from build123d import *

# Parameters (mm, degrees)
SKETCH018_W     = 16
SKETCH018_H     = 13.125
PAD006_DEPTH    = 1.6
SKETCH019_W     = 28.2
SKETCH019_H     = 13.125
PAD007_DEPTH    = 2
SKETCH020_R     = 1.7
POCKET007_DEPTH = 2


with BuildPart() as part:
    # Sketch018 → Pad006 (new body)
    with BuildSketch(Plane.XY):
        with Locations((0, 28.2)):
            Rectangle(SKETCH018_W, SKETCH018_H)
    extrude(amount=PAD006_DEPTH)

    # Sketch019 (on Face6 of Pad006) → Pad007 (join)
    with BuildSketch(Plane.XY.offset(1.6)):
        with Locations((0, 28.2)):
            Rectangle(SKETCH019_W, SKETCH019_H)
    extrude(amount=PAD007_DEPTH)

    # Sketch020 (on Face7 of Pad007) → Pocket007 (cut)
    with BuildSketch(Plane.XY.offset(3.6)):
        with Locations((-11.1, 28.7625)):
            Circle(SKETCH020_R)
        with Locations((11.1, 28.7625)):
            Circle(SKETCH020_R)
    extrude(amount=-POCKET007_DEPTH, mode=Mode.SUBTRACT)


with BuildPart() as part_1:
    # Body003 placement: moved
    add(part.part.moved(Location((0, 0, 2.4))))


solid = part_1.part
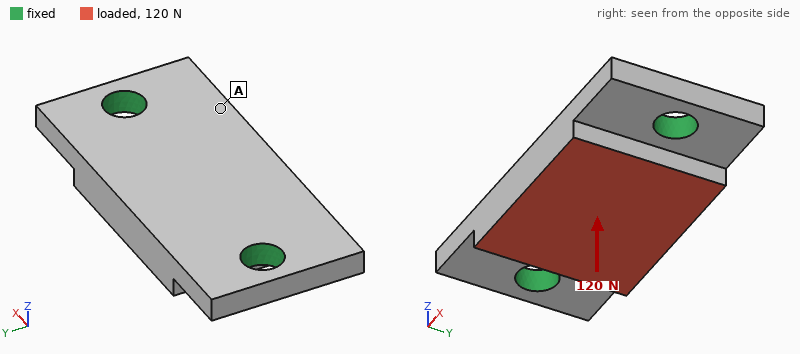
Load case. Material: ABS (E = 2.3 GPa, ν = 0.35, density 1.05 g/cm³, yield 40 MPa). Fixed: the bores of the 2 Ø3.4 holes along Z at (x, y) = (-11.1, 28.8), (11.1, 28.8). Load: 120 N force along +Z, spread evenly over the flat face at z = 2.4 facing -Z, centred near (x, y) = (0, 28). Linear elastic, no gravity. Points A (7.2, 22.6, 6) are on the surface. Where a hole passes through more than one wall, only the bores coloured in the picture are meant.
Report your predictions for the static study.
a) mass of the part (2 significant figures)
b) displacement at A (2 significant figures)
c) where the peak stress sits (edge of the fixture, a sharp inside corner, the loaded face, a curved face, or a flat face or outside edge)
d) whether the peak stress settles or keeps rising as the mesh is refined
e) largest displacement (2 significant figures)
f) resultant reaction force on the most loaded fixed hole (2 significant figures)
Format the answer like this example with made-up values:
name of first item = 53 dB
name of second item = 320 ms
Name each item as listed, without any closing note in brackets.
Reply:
mass of the part = 1.1 g
displacement at A = 0.066 mm
where the peak stress sits = edge of the fixture
whether the peak stress settles or keeps rising as the mesh is refined = keeps rising
largest displacement = 0.11 mm
resultant reaction force on the most loaded fixed hole = 77 N
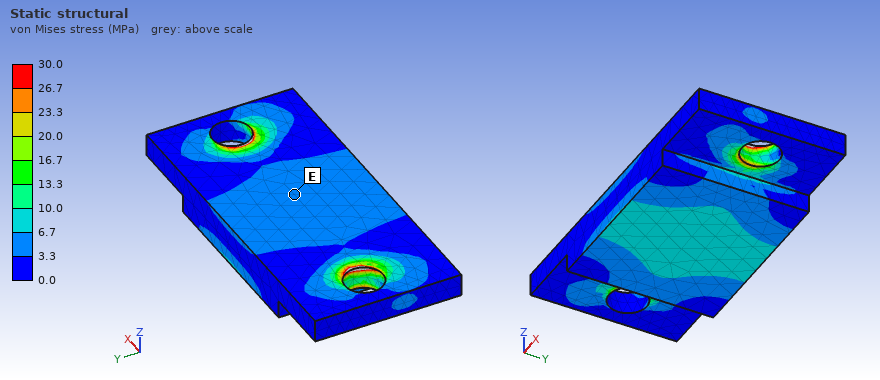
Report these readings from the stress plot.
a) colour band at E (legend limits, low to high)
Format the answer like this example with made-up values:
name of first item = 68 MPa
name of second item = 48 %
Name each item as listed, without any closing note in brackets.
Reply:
colour band at E = 3.3 to 6.7 MPa
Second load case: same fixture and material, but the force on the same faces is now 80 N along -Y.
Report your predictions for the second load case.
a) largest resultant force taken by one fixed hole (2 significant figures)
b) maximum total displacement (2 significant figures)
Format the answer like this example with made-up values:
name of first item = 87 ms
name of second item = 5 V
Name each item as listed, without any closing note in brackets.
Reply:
largest resultant force taken by one fixed hole = 40 N
maximum total displacement = 86 µm
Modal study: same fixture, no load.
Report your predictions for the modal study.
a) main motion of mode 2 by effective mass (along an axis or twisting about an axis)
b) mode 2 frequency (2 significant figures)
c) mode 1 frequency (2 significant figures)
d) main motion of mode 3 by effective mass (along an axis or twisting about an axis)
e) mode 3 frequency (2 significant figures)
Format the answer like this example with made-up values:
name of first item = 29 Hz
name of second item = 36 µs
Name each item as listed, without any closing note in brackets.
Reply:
main motion of mode 2 by effective mass = along Z
mode 2 frequency = 7600 Hz
mode 1 frequency = 6200 Hz
main motion of mode 3 by effective mass = along Y
mode 3 frequency = 14 kHz
